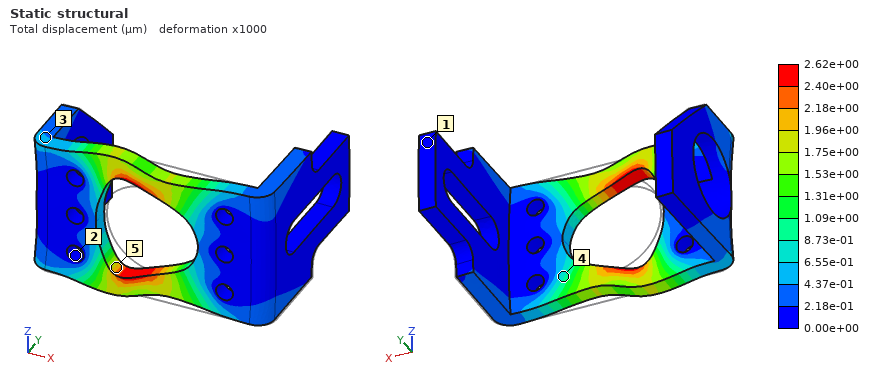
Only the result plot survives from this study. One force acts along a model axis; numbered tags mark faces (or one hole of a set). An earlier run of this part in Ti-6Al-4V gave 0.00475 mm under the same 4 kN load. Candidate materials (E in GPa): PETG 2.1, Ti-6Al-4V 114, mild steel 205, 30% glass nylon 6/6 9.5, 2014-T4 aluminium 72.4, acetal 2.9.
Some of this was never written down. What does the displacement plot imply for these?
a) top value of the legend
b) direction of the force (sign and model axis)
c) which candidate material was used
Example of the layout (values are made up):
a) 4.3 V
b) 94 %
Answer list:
a) 2.62e+00 µm
b) -X
c) mild steel
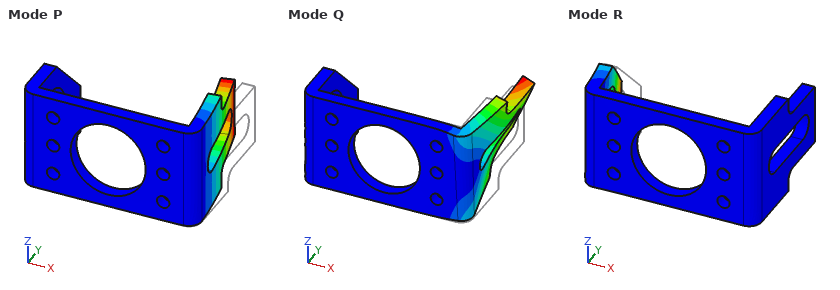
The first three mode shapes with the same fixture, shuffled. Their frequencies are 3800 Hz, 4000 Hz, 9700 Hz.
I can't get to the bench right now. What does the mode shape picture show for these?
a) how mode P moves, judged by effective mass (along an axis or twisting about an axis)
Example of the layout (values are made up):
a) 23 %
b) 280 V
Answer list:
a) along X
